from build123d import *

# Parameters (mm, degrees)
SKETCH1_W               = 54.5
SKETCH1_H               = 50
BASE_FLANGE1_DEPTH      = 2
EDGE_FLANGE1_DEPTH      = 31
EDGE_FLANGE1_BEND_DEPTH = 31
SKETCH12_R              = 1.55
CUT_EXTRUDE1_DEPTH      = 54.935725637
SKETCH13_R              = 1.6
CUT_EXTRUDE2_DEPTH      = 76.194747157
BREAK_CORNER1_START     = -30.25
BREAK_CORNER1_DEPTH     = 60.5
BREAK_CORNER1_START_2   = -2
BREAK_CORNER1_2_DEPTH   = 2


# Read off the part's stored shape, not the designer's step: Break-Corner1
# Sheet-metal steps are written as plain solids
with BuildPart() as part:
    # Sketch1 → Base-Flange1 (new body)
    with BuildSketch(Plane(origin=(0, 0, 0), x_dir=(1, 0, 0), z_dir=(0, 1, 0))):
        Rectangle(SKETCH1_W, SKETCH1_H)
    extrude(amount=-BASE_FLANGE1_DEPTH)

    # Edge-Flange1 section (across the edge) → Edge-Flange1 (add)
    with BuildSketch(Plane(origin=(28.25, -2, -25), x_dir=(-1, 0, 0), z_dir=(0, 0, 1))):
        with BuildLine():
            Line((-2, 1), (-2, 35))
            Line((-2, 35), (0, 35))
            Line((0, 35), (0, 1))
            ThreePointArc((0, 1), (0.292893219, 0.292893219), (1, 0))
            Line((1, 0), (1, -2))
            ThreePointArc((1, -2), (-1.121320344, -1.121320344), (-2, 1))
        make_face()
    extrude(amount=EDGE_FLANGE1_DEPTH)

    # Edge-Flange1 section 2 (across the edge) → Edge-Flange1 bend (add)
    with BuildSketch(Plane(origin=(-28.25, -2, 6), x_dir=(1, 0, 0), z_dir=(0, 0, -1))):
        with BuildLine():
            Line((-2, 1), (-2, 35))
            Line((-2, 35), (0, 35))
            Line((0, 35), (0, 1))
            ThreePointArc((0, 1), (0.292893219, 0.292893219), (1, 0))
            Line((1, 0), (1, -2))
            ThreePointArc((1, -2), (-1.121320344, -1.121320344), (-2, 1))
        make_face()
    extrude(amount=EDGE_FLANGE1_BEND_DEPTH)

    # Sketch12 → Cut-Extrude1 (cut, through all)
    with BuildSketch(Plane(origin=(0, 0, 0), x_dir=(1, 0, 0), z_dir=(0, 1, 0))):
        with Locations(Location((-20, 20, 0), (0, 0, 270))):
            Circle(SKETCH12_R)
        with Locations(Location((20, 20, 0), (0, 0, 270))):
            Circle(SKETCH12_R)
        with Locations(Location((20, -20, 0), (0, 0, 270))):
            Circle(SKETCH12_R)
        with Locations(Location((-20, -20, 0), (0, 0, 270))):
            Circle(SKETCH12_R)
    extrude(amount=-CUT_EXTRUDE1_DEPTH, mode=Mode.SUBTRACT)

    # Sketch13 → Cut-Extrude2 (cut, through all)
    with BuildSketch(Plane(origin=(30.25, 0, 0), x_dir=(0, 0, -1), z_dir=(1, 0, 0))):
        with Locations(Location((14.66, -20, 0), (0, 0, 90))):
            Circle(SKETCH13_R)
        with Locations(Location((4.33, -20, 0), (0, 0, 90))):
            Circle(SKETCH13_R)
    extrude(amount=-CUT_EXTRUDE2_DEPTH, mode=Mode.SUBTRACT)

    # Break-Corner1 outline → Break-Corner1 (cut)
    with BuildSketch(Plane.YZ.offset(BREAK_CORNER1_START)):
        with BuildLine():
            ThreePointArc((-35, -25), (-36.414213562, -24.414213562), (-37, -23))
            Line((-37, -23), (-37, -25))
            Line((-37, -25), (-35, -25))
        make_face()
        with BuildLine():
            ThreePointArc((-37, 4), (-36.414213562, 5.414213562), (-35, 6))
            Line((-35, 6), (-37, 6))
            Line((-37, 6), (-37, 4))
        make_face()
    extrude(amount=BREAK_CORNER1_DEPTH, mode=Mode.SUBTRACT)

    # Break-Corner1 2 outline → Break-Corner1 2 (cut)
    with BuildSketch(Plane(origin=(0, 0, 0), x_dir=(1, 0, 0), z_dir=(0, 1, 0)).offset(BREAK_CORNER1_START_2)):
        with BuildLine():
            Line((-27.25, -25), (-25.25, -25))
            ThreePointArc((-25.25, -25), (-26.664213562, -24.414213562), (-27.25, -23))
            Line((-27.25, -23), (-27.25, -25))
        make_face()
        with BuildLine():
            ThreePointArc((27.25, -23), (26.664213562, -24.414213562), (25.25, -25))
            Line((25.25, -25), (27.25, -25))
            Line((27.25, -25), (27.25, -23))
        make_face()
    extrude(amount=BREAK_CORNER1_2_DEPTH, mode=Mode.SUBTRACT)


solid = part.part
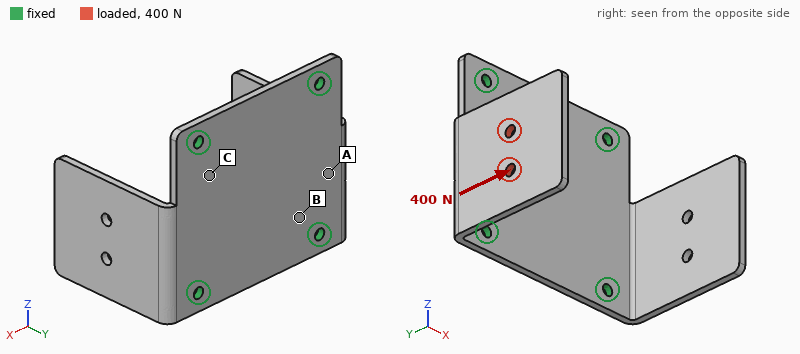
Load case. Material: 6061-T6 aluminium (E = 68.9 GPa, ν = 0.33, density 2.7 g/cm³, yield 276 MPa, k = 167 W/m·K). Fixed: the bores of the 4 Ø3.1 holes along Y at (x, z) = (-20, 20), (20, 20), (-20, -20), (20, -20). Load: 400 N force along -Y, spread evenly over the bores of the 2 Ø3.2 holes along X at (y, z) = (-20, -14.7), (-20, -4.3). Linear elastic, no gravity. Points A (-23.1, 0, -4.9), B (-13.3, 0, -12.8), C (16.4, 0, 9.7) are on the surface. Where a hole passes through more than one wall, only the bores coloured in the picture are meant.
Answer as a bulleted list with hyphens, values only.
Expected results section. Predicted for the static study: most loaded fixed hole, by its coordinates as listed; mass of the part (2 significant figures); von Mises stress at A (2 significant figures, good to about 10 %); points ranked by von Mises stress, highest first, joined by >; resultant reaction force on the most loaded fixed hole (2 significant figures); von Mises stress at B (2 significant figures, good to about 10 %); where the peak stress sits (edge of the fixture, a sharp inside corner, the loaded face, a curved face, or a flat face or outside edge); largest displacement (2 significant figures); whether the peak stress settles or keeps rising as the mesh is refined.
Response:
- (-20, -20)
- 27 g
- 45 MPa
- A > B > C
- 310 N
- 29 MPa
- edge of the fixture
- 0.56 mm
- keeps rising
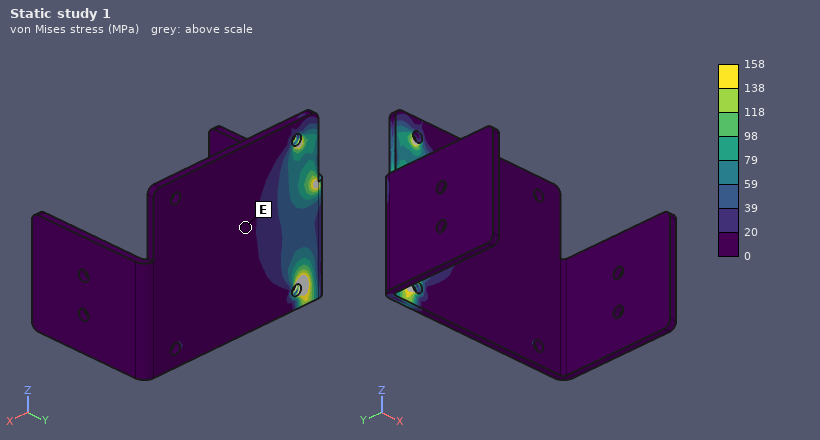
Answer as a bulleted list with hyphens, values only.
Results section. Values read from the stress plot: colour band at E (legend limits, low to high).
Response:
- 0 to 20 MPa
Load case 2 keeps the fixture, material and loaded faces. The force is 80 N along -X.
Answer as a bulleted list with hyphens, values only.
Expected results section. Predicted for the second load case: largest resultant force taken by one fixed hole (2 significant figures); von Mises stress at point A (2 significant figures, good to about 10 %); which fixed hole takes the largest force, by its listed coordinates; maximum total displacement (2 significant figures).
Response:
- 43 N
- 44 MPa
- (-20, -20)
- 0.62 mm
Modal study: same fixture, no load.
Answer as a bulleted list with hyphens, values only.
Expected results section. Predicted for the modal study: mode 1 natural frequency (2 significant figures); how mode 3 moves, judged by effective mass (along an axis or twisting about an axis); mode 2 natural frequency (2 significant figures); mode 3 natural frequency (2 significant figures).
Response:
- 900 Hz
- along Z
- 910 Hz
- 2200 Hz
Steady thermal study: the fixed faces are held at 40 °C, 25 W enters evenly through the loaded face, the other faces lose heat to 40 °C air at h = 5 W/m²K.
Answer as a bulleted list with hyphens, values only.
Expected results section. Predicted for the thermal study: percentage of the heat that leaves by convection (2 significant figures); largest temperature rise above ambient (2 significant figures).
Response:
- 3.7 %
- 81 K
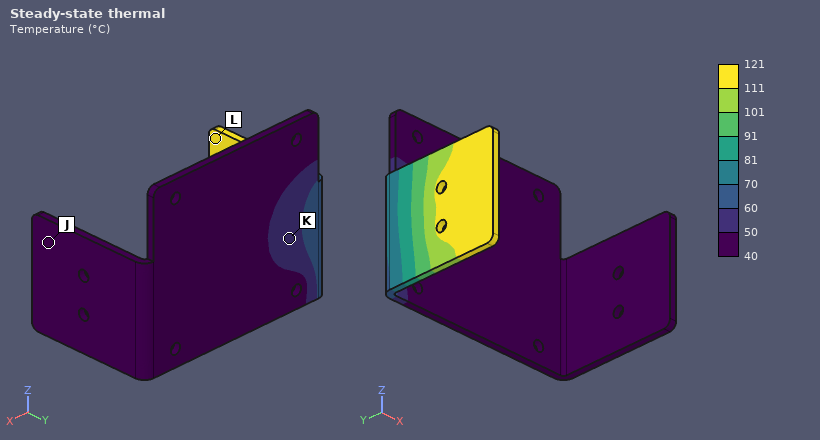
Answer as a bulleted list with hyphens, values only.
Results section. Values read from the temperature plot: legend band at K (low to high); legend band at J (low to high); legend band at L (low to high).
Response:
- 50 to 60 °C
- 40 to 50 °C
- 111 to 121 °C
